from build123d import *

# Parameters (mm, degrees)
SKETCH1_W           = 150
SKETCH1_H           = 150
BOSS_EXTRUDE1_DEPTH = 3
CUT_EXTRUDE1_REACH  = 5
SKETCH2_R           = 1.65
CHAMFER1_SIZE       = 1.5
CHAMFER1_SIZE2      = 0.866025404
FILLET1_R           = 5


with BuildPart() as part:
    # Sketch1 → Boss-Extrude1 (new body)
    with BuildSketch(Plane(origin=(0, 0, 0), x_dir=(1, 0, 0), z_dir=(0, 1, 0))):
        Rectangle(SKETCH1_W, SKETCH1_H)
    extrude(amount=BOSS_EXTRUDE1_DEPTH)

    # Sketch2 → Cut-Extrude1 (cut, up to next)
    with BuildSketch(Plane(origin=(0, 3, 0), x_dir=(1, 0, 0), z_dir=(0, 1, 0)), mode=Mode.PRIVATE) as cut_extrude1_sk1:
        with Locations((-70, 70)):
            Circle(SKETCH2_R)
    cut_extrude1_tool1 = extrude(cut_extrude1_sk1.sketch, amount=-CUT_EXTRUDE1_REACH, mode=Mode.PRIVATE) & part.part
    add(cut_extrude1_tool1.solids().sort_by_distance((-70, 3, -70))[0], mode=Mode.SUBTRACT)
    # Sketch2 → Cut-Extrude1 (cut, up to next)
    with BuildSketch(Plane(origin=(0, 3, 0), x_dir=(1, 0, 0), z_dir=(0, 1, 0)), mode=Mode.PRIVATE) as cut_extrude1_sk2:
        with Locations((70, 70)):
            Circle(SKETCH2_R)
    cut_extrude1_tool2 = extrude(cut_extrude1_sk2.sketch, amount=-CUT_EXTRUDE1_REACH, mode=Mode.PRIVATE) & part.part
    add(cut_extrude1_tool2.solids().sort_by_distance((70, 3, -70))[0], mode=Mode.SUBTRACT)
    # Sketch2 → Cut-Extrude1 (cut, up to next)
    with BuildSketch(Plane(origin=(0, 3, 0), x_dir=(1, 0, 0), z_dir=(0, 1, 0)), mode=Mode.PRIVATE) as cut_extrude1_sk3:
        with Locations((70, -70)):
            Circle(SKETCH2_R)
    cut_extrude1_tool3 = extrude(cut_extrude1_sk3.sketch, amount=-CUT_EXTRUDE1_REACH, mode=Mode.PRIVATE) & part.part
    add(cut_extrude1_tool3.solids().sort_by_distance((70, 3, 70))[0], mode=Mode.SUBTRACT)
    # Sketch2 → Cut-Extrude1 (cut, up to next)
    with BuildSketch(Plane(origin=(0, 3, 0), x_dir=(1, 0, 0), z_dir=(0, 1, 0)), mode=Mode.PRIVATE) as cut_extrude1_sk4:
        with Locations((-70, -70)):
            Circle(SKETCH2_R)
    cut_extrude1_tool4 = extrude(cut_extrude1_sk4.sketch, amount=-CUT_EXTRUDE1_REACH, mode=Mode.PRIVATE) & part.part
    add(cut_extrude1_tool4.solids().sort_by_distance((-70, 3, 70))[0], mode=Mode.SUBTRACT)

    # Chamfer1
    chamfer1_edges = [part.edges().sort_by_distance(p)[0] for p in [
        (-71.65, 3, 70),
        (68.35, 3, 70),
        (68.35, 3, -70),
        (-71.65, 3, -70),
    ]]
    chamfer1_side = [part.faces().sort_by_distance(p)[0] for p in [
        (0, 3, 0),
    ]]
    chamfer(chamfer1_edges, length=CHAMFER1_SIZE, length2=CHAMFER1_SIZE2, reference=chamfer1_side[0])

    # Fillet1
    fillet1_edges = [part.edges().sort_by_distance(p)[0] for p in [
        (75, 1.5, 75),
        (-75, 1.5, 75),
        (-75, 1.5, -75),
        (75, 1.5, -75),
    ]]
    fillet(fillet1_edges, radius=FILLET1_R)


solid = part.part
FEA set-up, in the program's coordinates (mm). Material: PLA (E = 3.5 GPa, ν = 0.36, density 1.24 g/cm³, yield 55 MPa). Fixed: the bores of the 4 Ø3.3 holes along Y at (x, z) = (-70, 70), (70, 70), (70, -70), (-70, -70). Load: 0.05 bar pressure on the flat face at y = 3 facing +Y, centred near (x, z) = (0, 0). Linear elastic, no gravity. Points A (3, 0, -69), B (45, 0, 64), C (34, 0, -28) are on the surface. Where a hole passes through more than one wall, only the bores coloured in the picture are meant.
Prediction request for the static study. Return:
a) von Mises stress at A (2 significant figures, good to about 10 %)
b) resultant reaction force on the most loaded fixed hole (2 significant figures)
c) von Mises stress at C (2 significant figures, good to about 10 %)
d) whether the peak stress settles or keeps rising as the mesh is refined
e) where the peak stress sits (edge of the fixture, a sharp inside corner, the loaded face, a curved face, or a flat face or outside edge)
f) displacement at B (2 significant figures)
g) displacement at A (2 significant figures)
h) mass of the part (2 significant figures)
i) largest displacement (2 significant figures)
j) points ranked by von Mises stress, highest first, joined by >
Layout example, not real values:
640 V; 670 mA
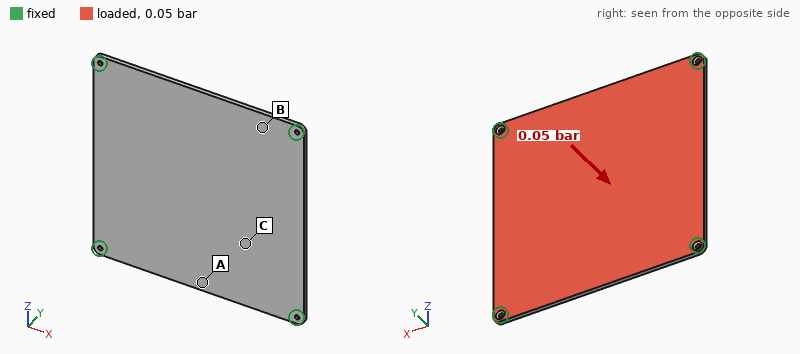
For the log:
4.8 MPa; 36 N; 3.3 MPa; keeps rising; edge of the fixture; 0.66 mm; 1.4 mm; 83 g; 2.3 mm; A > C > B
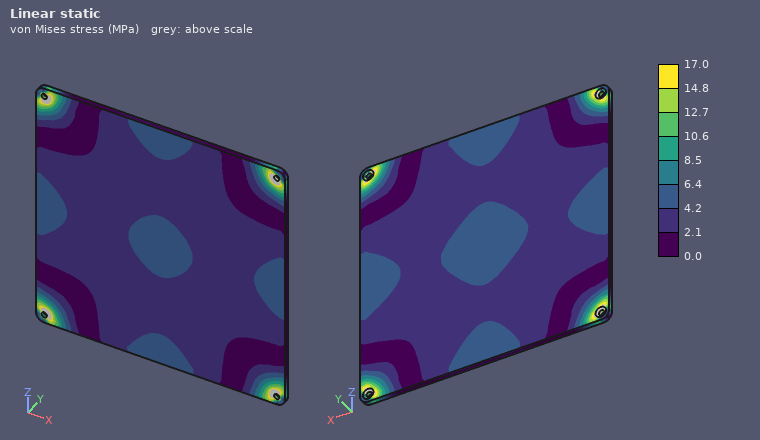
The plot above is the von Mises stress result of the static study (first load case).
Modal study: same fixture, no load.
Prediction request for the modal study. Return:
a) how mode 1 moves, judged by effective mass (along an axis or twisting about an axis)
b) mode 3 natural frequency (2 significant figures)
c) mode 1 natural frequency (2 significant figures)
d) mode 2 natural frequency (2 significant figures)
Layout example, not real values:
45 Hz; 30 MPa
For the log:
along Y; 270 Hz; 150 Hz; 270 Hz
